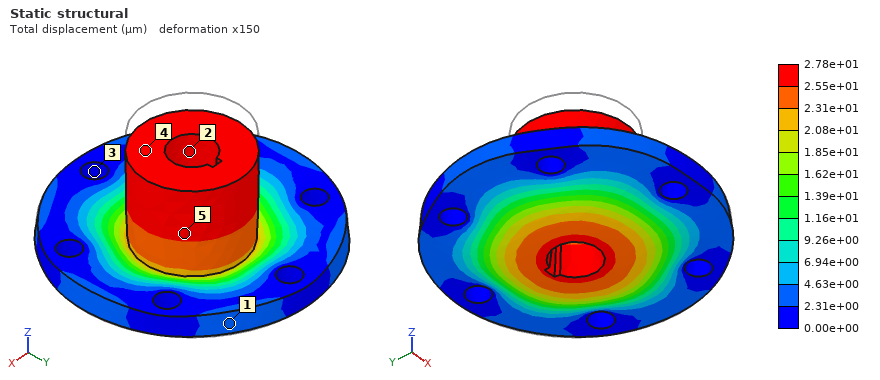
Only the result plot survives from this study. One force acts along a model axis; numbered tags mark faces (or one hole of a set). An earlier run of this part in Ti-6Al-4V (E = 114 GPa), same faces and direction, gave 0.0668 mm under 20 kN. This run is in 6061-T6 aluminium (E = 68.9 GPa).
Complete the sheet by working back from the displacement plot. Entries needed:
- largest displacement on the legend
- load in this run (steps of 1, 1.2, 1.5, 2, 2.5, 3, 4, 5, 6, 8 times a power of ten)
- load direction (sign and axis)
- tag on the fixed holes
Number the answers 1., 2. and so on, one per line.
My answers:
1. 2.78e+01 µm
2. 5 kN
3. -Z
4. 3
